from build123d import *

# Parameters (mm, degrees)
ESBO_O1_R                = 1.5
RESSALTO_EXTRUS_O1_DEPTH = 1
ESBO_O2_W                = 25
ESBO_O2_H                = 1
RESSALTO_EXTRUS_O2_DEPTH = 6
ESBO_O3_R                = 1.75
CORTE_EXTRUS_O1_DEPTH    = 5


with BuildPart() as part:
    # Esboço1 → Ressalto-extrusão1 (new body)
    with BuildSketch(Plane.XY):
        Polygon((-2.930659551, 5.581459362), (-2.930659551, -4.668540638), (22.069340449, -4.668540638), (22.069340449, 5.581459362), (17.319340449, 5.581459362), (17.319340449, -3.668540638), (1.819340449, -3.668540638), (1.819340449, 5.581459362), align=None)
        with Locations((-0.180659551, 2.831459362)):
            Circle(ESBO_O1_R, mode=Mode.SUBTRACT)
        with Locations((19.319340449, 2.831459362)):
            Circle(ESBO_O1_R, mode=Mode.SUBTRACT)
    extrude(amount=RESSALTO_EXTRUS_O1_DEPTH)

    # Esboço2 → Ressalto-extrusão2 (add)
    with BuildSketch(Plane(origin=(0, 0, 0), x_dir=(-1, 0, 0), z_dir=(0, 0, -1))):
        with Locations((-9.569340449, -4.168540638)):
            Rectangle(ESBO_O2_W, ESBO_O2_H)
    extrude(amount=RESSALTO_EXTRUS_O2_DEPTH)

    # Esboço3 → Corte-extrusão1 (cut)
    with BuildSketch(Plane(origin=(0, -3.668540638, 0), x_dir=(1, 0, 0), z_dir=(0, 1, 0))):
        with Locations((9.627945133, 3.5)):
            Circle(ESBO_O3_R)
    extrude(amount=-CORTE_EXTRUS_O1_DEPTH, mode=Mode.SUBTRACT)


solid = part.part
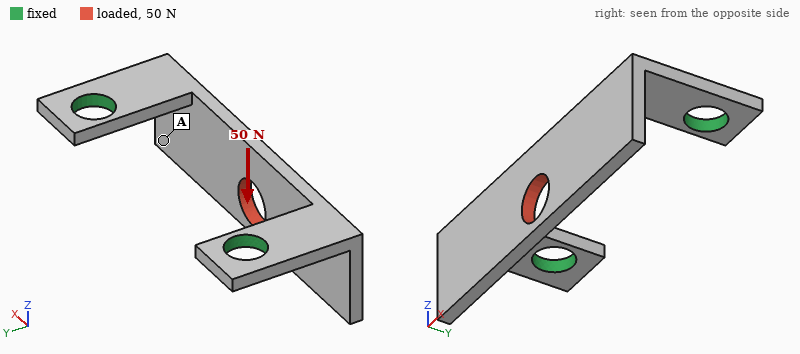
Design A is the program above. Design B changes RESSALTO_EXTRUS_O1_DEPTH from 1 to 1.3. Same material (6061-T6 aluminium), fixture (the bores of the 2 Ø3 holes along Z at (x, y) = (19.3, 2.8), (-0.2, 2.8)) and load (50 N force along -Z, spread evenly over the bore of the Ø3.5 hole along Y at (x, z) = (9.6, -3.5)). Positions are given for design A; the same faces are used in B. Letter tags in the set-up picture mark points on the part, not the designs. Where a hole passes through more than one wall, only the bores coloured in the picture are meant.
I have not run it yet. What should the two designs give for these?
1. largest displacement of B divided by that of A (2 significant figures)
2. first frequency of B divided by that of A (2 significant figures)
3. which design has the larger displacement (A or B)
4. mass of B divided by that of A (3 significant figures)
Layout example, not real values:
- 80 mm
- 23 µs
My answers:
- 0.49
- 1.4
- A
- 1.12
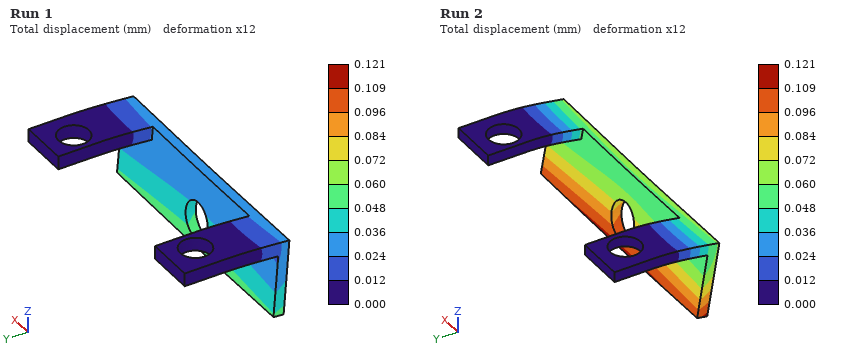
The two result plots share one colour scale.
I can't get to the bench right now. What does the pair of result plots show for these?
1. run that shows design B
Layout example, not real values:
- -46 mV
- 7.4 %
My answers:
- Run 1
